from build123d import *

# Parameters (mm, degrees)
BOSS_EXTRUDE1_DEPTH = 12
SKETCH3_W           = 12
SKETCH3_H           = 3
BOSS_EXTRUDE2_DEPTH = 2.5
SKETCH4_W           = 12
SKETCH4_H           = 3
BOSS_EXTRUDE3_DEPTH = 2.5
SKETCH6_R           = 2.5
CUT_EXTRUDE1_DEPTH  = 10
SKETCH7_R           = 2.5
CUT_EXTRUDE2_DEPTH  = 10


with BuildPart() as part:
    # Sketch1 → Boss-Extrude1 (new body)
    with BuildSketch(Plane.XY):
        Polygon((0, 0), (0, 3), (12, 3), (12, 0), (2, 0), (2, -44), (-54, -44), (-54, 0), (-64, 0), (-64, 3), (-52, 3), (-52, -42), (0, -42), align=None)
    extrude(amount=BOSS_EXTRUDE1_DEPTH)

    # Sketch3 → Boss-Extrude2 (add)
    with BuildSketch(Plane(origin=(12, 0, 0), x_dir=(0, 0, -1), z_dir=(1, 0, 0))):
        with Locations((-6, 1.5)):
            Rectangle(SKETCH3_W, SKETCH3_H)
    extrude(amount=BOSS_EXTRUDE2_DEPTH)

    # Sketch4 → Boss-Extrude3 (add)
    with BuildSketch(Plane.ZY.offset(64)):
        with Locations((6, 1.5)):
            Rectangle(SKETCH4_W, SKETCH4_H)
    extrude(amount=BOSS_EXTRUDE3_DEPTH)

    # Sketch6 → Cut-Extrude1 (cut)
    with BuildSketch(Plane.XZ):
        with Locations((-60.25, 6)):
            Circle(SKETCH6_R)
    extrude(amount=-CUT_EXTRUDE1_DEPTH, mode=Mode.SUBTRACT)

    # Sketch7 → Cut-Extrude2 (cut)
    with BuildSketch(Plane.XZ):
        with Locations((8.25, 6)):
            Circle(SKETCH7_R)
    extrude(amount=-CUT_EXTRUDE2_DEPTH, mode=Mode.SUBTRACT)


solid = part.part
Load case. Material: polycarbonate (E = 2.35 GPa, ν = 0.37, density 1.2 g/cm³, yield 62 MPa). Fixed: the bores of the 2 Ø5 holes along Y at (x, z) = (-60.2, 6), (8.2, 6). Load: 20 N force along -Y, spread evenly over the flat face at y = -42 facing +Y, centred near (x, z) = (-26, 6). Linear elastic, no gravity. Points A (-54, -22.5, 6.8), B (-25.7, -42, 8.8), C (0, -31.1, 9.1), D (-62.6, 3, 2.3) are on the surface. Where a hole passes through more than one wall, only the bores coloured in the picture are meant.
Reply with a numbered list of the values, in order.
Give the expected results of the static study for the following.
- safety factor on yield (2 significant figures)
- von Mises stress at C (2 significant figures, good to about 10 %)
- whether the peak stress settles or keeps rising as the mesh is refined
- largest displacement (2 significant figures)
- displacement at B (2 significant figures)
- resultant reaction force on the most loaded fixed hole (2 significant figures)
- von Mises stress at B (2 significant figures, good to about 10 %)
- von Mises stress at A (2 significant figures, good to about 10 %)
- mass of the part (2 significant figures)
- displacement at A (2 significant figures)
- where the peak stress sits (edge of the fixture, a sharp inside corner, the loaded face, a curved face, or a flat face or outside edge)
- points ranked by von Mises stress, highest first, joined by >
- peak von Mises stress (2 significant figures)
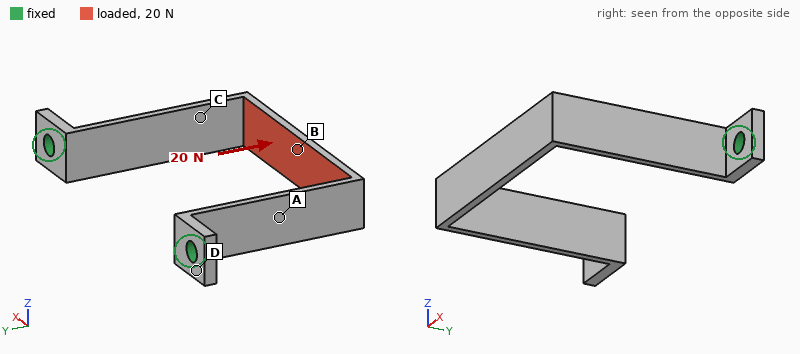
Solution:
1. 6.9
2. 5.4 MPa
3. settles
4. 0.95 mm
5. 0.93 mm
6. 10 N
7. 8.7 MPa
8. 2.1 MPa
9. 5.1 g
10. 0.23 mm
11. a flat face or outside edge
12. B > C > A > D
13. 9.0 MPa
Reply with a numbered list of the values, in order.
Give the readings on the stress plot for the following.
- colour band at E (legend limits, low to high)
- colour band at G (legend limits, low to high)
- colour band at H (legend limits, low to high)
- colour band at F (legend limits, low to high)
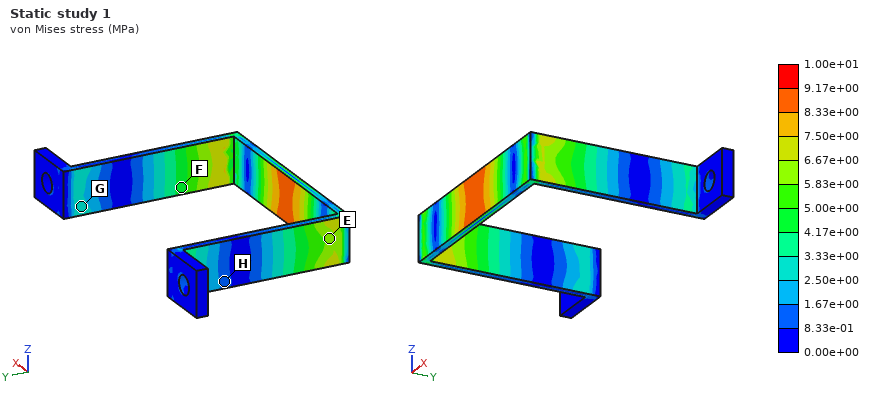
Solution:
1. 5.83e+00 to 6.67e+00 MPa
2. 2.50e+00 to 3.33e+00 MPa
3. 8.33e-01 to 1.67e+00 MPa
4. 4.17e+00 to 5.00e+00 MPa
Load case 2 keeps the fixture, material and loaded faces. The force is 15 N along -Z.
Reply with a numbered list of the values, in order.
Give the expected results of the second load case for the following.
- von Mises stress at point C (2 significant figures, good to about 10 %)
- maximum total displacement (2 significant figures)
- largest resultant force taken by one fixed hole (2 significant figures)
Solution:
1. 1.6 MPa
2. 1.1 mm
3. 7.5 N
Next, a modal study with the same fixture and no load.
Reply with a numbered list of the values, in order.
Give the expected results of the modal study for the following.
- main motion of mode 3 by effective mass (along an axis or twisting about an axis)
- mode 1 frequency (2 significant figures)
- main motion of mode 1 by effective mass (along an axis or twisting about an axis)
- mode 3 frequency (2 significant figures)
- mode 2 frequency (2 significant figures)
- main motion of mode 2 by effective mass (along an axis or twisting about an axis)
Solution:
1. twisting about Y
2. 190 Hz
3. along X
4. 550 Hz
5. 380 Hz
6. along Z
